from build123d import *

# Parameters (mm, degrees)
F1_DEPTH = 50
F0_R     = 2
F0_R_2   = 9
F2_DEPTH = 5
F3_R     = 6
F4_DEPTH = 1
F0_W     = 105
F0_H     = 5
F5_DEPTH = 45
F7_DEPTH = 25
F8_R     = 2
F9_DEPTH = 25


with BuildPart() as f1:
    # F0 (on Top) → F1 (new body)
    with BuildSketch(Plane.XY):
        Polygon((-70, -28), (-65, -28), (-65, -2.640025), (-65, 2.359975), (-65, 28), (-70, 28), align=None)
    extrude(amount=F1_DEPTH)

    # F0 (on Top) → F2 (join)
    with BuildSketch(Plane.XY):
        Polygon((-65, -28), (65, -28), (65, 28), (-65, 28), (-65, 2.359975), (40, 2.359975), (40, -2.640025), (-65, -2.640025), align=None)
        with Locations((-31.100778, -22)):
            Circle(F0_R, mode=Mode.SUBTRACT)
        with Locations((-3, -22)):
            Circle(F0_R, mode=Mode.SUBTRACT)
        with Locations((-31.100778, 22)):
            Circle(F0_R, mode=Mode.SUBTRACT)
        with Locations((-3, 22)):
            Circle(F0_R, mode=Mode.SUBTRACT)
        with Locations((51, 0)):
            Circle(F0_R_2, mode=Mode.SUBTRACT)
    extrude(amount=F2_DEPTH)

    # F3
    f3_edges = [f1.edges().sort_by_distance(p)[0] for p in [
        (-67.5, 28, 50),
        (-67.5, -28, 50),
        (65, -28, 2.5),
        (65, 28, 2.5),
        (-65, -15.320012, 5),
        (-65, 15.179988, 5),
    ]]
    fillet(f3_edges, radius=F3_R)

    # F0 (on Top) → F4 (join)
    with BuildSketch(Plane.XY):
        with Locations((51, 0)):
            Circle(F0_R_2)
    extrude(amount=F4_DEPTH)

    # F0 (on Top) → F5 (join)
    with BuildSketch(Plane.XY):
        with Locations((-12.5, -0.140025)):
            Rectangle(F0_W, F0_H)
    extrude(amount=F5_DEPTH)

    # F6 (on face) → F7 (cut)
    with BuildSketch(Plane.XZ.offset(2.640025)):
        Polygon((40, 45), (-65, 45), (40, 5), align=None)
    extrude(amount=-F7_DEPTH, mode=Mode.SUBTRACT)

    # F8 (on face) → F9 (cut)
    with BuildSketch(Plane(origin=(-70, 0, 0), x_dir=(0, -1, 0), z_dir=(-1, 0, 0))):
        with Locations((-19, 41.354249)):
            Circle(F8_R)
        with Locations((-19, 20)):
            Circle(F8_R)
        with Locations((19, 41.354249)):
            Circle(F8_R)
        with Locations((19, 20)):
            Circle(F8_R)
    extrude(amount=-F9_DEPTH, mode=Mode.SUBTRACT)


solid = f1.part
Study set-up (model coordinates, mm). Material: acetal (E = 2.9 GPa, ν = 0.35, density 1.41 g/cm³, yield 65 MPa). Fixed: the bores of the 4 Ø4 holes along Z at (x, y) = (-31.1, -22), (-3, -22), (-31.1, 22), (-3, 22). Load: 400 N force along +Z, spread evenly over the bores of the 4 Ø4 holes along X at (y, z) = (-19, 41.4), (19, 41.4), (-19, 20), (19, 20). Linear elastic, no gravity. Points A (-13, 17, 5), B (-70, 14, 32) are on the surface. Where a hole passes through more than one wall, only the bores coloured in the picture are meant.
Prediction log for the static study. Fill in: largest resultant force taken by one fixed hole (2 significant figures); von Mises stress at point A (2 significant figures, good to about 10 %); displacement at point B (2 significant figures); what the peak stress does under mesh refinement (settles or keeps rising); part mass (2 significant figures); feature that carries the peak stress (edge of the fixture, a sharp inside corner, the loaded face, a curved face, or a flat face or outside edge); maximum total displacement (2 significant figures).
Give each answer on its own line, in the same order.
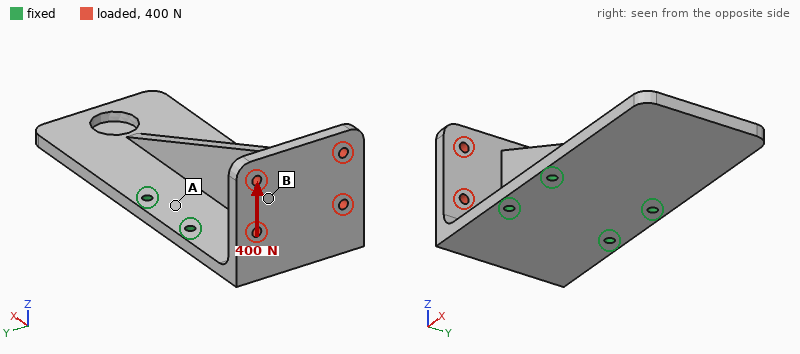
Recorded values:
380 N
6.2 MPa
1.3 mm
keeps rising
84 g
edge of the fixture
1.5 mm
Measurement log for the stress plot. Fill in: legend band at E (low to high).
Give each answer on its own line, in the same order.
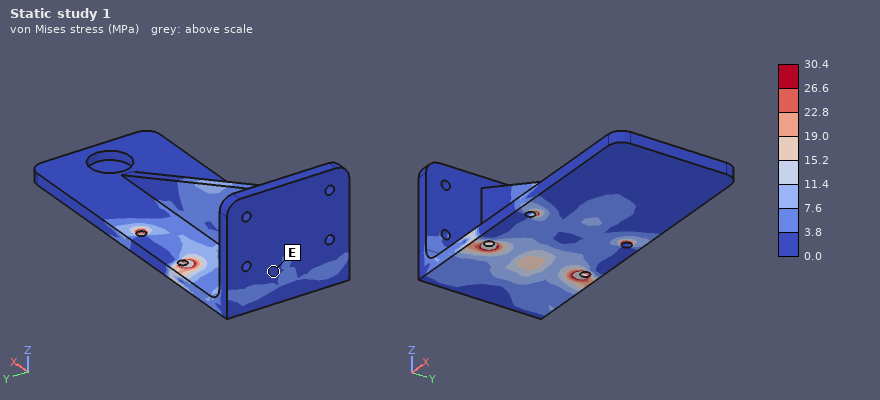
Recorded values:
0.0 to 3.8 MPa
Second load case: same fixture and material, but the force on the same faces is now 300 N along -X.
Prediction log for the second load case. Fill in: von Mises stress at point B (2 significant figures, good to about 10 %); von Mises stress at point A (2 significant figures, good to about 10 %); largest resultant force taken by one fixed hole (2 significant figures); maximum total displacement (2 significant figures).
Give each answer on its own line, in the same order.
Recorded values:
3.5 MPa
3.5 MPa
140 N
0.94 mm
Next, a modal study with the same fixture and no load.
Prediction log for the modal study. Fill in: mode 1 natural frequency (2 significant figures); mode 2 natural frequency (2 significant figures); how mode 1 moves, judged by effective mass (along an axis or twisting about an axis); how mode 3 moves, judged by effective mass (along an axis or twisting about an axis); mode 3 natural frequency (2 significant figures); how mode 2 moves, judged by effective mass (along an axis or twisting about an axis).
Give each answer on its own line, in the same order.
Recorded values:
380 Hz
510 Hz
twisting about Y
along Z
630 Hz
along Y
